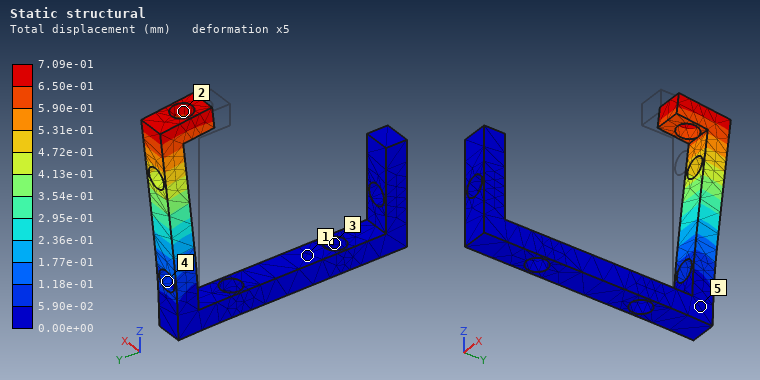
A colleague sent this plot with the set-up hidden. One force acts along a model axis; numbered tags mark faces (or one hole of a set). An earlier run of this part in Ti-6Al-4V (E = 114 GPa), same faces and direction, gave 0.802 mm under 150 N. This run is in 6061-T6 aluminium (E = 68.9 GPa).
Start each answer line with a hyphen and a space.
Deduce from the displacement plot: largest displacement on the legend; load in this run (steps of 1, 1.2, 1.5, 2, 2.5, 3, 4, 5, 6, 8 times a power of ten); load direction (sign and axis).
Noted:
- 7.09e-01 mm
- 80 N
- +Y
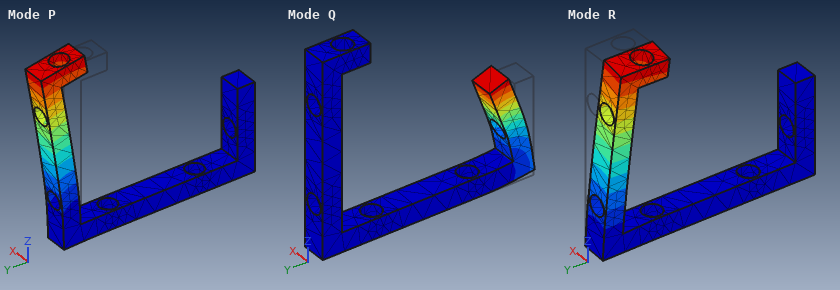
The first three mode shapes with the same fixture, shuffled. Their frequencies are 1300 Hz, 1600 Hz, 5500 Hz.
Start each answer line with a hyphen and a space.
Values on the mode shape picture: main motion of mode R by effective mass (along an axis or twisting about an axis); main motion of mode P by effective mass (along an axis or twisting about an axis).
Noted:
- along X
- along Y
